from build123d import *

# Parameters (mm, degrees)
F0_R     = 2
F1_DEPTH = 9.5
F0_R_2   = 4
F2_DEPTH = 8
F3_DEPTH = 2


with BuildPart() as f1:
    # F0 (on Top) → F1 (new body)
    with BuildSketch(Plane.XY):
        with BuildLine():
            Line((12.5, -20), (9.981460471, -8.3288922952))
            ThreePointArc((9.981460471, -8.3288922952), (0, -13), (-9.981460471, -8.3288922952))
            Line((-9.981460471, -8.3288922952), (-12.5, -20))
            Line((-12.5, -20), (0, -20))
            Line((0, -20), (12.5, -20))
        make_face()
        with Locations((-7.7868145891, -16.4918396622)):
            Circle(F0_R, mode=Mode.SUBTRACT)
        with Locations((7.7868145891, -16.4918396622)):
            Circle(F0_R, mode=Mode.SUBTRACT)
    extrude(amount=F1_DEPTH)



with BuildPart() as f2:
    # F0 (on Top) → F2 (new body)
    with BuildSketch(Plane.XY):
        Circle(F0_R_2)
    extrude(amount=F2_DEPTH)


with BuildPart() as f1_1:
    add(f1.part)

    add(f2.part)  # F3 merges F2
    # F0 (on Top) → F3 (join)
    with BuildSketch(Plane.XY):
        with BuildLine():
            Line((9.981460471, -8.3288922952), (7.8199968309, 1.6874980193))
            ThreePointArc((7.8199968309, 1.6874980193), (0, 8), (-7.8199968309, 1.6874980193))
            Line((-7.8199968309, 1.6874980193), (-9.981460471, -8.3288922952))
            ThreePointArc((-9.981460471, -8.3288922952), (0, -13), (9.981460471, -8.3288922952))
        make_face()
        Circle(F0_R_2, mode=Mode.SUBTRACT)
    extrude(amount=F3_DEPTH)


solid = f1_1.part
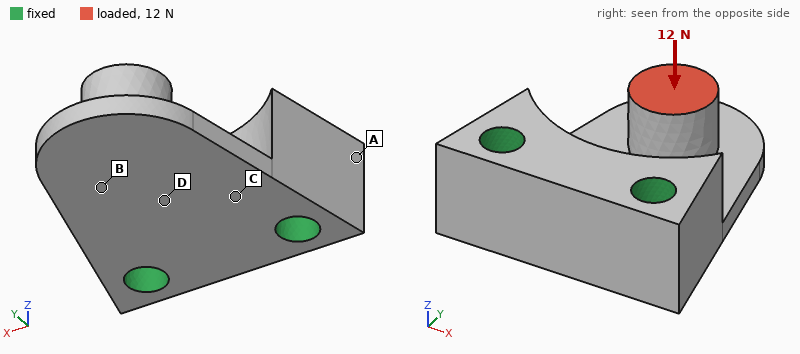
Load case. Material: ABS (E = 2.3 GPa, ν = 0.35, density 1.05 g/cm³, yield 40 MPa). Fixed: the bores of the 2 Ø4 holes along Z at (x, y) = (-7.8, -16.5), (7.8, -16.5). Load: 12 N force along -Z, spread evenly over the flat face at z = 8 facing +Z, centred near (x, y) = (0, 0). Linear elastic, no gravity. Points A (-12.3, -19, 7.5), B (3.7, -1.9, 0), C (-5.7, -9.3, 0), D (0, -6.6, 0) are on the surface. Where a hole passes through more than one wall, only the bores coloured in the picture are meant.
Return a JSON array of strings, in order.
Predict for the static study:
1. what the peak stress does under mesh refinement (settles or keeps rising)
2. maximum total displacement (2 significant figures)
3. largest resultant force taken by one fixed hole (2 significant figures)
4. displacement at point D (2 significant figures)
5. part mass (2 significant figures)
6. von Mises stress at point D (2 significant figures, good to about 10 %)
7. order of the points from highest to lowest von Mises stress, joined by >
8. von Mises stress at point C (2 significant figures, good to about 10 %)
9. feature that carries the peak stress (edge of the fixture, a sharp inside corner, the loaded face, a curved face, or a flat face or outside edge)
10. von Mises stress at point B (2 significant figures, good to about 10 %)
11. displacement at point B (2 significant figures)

["keeps rising", "0.45 mm", "6.1 N", "0.074 mm", "2.7 g", "5.1 MPa", "C > D > B > A", "7.3 MPa", "a sharp inside corner", "2.7 MPa", "0.18 mm"]
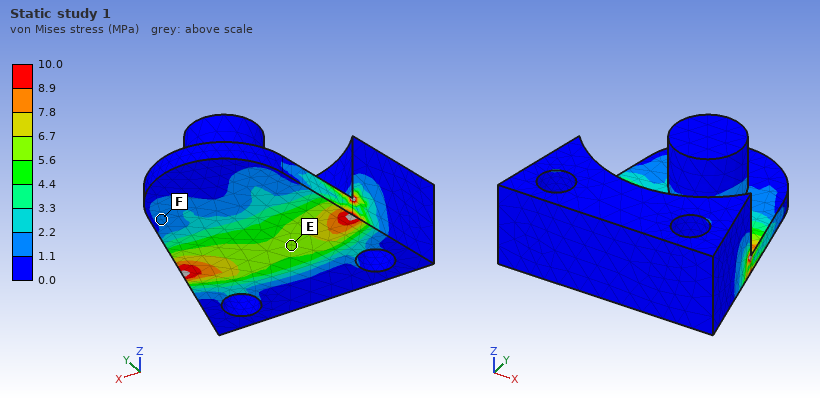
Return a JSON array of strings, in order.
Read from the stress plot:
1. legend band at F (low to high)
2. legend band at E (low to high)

["1.1 to 2.2 MPa", "5.6 to 6.7 MPa"]
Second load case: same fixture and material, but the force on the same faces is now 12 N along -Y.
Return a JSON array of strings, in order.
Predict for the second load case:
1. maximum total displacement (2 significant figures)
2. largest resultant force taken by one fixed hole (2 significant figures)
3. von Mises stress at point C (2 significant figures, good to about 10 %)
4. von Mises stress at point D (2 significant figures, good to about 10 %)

["0.40 mm", "6.4 N", "5.1 MPa", "5.6 MPa"]
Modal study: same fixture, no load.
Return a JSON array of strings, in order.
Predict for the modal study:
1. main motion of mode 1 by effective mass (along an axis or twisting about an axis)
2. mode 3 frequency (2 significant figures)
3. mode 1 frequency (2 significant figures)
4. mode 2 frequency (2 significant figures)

["along Z", "6100 Hz", "1200 Hz", "3800 Hz"]
